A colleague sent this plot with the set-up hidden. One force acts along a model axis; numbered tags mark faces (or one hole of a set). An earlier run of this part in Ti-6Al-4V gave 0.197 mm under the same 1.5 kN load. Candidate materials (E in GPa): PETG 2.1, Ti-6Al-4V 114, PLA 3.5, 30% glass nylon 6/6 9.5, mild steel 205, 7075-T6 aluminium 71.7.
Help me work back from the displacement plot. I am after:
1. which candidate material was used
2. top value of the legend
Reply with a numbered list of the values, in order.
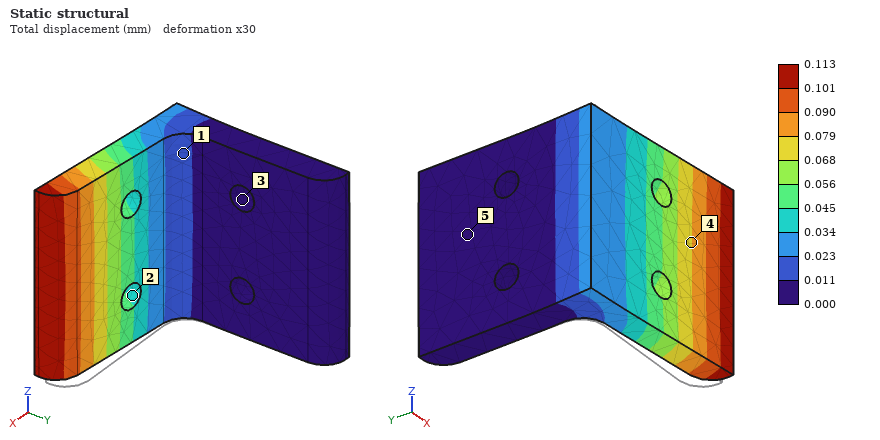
1. mild steel
2. 0.113 mm
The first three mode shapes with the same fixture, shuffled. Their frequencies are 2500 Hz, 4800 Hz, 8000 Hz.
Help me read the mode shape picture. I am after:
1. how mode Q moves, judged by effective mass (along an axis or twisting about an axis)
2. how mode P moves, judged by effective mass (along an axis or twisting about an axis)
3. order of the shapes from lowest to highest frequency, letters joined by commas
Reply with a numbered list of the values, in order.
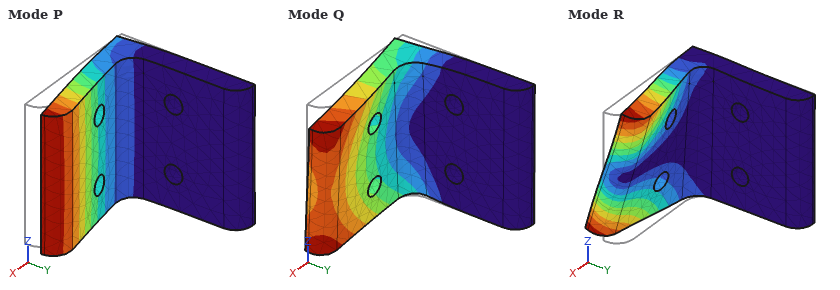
1. along Z
2. along Y
3. P, Q, R
